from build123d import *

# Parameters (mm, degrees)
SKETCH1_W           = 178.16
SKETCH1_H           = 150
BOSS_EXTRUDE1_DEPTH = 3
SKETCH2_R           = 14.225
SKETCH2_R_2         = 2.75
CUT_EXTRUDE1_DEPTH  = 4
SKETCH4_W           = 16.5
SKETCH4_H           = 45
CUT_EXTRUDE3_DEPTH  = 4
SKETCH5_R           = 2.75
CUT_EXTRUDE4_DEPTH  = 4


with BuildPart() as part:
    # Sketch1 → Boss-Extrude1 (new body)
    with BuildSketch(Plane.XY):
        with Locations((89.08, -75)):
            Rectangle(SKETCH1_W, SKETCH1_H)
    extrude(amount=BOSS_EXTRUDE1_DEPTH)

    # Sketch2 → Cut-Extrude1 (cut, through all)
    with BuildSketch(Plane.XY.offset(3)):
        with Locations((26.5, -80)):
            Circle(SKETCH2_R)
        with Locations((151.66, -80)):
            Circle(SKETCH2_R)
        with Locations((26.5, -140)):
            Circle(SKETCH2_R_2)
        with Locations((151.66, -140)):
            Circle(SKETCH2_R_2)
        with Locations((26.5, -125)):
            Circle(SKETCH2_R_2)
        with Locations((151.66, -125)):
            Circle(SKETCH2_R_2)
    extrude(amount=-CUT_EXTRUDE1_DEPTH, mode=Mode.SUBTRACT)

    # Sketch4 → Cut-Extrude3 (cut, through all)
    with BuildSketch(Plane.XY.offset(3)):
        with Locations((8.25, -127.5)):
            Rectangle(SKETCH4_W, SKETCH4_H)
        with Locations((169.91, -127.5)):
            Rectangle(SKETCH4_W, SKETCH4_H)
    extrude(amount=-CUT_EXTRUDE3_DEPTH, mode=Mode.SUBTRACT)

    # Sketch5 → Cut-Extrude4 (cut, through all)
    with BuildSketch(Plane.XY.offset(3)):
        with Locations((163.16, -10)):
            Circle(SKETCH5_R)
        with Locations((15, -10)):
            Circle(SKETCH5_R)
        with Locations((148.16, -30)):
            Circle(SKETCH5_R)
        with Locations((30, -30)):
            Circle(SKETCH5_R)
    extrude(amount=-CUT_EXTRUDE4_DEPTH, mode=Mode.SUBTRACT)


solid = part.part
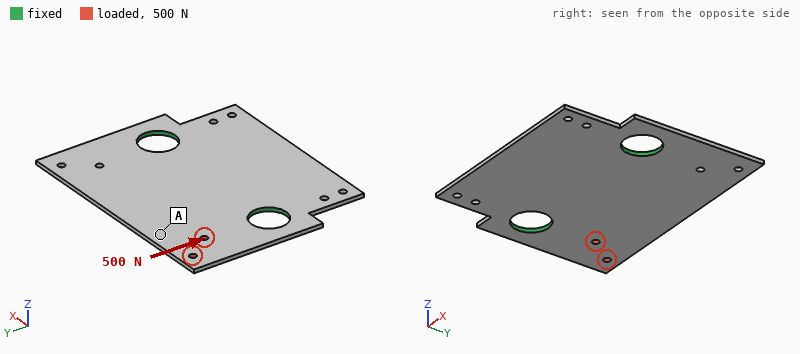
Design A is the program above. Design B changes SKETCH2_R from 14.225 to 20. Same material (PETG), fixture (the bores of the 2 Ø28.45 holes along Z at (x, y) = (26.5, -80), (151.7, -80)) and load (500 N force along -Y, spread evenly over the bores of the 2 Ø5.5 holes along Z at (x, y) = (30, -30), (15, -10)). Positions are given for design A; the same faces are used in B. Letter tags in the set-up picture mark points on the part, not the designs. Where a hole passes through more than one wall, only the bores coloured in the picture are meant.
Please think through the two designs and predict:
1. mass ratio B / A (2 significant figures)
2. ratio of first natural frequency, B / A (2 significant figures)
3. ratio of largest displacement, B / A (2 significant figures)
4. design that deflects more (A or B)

0.95
1.2
0.89
A
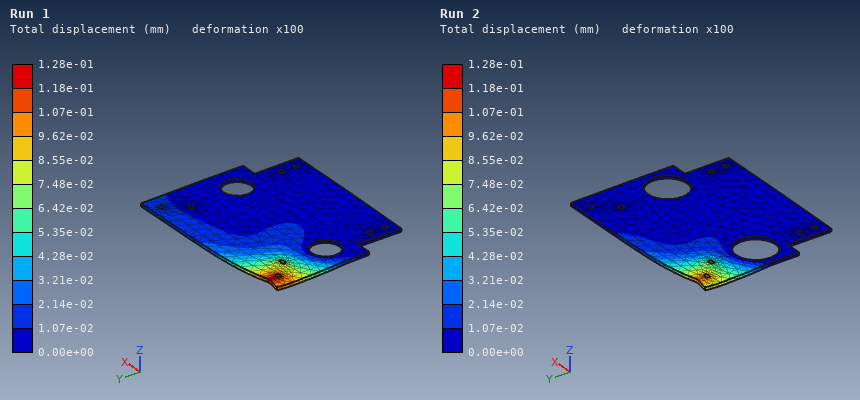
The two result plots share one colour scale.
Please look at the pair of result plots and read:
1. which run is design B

Run 2
